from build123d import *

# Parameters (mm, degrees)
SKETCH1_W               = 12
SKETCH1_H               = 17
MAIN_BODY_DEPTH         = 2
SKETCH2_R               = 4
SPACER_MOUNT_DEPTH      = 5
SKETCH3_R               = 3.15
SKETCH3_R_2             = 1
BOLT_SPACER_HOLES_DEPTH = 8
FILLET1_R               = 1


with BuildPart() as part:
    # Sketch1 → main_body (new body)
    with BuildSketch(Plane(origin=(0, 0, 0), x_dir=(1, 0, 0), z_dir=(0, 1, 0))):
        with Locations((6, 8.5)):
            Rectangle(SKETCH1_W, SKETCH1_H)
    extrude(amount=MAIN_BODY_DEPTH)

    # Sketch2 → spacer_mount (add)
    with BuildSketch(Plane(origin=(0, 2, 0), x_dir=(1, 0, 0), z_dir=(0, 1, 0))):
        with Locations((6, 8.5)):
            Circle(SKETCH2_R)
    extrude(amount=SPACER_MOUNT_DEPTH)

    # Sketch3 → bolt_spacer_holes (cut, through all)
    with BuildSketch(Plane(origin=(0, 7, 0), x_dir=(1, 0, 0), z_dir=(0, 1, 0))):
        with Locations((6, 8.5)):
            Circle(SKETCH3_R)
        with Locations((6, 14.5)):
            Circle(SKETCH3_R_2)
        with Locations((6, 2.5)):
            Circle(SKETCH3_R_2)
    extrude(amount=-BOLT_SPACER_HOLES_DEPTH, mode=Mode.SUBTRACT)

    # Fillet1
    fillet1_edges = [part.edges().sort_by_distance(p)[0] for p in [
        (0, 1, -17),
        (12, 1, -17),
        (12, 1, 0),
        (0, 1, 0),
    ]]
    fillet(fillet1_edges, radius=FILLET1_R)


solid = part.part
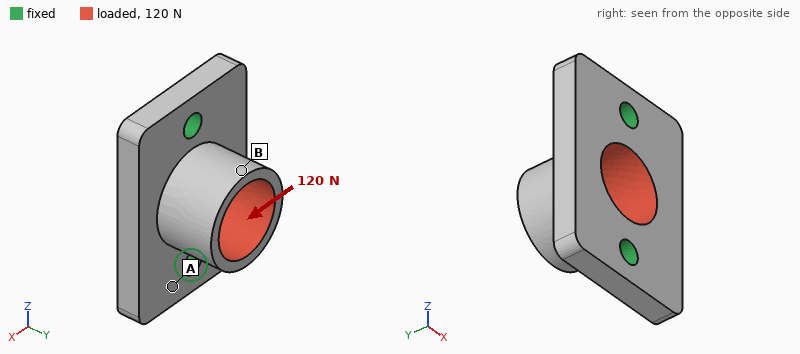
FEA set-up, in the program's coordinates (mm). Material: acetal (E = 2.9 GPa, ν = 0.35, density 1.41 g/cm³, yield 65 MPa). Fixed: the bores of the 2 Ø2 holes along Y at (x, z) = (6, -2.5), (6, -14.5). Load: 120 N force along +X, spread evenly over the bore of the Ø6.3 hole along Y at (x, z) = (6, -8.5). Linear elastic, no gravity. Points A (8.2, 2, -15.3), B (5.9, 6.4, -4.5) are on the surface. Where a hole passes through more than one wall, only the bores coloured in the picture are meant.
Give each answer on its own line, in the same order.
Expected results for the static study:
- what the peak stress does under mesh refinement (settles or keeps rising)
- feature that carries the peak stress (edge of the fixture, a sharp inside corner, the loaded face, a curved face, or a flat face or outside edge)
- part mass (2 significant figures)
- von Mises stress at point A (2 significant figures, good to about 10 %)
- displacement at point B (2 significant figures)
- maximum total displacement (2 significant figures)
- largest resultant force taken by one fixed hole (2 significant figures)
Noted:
keeps rising
edge of the fixture
0.60 g
11 MPa
0.12 mm
0.16 mm
60 N
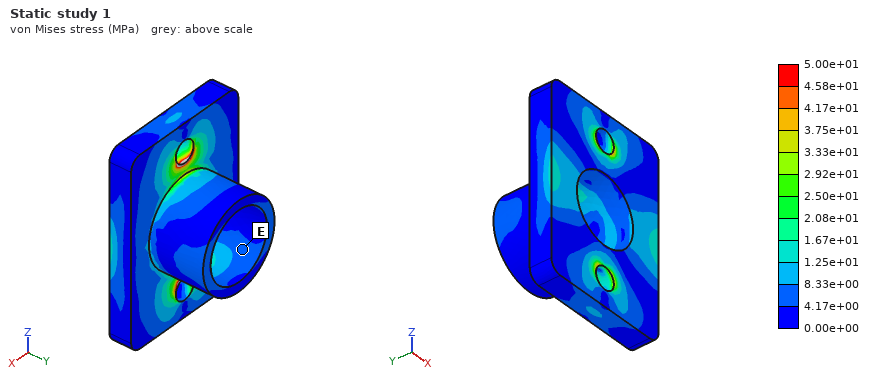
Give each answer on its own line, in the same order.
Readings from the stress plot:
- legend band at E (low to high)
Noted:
4.17e+00 to 8.33e+00 MPa
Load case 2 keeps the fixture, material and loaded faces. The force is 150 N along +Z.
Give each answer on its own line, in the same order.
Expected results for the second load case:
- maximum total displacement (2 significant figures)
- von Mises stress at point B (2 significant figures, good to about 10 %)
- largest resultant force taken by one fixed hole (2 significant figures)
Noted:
62 µm
4.2 MPa
84 N
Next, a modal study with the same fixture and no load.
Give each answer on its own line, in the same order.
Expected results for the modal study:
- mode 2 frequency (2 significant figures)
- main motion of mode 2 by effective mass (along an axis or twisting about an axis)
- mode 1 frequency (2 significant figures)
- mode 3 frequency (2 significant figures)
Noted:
12 kHz
along Y
8100 Hz
15 kHz
